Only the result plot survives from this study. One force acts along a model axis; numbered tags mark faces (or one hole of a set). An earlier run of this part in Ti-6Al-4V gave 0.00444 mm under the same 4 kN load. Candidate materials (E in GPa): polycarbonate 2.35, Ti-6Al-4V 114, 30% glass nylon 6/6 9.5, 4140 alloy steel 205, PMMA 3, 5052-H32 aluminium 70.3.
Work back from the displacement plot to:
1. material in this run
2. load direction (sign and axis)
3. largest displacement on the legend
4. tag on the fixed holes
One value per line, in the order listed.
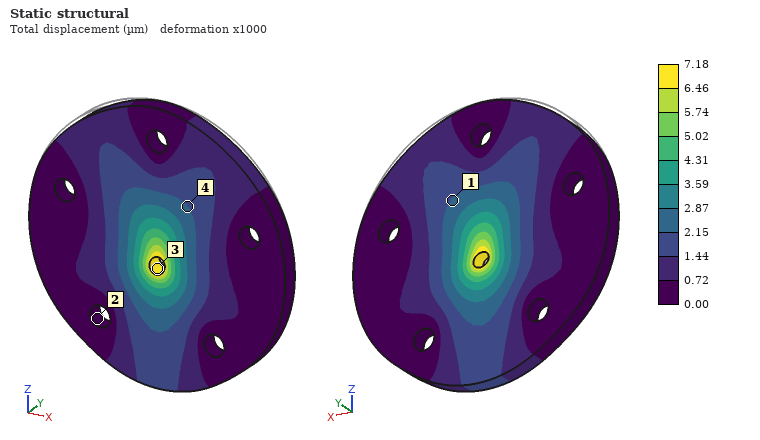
5052-H32 aluminium
-Z
7.18 µm
2
